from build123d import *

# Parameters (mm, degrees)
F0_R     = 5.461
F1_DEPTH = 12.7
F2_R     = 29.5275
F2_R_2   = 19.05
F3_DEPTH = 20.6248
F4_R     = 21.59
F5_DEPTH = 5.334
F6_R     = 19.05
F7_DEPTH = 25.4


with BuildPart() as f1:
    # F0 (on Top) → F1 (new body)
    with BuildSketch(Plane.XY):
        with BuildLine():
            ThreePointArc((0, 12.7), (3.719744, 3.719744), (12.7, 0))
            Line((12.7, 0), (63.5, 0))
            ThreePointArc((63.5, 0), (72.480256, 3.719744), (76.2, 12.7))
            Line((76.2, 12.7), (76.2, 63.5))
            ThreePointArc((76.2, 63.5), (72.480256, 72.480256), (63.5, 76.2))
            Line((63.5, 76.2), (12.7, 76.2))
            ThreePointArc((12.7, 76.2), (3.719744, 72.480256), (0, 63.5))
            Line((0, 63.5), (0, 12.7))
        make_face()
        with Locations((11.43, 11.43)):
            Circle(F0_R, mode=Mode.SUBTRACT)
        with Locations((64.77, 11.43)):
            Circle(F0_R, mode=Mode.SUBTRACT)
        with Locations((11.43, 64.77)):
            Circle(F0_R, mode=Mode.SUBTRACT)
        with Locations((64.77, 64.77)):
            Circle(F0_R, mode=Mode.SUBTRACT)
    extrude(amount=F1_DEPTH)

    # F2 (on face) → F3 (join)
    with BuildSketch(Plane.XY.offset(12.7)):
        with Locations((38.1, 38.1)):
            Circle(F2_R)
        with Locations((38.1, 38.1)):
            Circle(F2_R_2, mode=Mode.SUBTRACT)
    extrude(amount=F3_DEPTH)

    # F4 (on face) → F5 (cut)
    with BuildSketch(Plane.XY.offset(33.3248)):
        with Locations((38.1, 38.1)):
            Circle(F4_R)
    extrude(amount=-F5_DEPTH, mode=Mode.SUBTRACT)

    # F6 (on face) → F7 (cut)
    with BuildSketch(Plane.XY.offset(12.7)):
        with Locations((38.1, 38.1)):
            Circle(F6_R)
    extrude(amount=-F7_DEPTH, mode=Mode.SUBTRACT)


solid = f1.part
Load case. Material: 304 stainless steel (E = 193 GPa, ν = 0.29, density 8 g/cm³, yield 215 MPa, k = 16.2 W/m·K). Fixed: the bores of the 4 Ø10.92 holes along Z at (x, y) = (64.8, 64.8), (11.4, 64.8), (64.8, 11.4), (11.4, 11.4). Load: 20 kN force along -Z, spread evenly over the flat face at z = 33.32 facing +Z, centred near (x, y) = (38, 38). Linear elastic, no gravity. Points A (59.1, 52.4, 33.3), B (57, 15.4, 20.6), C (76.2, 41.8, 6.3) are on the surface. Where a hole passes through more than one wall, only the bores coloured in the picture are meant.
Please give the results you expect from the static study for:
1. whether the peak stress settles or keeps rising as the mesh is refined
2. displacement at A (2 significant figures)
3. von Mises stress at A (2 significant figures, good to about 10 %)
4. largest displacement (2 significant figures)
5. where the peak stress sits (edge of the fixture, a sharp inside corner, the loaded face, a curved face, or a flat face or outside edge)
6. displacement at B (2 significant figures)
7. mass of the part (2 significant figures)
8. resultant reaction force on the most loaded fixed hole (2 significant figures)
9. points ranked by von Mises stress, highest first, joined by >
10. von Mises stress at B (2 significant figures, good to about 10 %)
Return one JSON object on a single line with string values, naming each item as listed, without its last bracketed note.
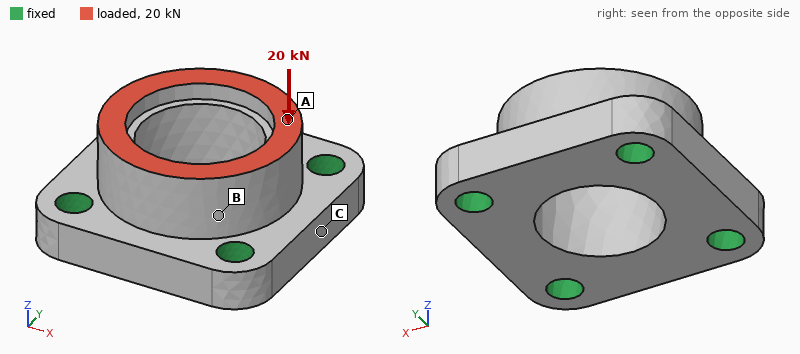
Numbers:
{"whether the peak stress settles or keeps rising as the mesh is refined": "keeps rising", "displacement at A": "4.4 µm", "von Mises stress at A": "17 MPa", "largest displacement": "4.9 µm", "where the peak stress sits": "edge of the fixture", "displacement at B": "3.5 µm", "mass of the part": "670 g", "resultant reaction force on the most loaded fixed hole": "5.2 kN", "points ranked by von Mises stress, highest first, joined by >": "B > A > C", "von Mises stress at B": "23 MPa"}
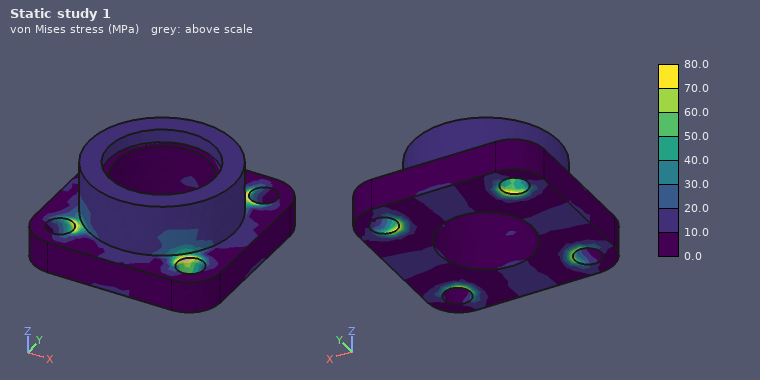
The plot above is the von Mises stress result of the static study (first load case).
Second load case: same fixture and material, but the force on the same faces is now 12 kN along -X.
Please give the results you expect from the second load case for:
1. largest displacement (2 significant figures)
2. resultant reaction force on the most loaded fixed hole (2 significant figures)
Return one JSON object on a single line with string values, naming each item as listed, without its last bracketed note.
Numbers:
{"largest displacement": "12 µm", "resultant reaction force on the most loaded fixed hole": "4.4 kN"}
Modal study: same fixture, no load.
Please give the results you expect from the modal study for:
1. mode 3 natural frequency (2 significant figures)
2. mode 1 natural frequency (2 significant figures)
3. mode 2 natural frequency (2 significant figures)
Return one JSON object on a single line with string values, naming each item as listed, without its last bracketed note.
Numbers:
{"mode 3 natural frequency": "17 kHz", "mode 1 natural frequency": "15 kHz", "mode 2 natural frequency": "17 kHz"}
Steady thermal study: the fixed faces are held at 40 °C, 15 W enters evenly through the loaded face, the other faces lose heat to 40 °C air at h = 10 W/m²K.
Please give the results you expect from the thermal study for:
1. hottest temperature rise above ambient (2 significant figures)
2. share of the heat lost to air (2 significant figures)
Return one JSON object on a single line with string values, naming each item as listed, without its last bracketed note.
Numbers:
{"hottest temperature rise above ambient": "20 K", "share of the heat lost to air": "8.3 %"}
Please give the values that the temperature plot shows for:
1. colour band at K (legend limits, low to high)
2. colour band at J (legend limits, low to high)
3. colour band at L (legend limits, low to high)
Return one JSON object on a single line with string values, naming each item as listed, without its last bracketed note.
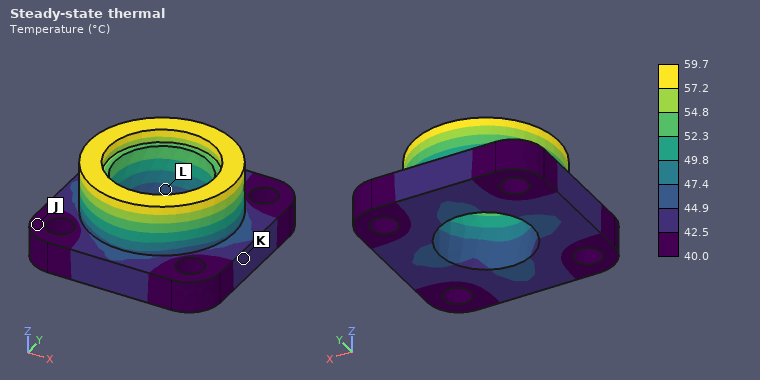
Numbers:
{"colour band at K": "42.5 to 44.9 °C", "colour band at J": "40.0 to 42.5 °C", "colour band at L": "44.9 to 47.4 °C"}
